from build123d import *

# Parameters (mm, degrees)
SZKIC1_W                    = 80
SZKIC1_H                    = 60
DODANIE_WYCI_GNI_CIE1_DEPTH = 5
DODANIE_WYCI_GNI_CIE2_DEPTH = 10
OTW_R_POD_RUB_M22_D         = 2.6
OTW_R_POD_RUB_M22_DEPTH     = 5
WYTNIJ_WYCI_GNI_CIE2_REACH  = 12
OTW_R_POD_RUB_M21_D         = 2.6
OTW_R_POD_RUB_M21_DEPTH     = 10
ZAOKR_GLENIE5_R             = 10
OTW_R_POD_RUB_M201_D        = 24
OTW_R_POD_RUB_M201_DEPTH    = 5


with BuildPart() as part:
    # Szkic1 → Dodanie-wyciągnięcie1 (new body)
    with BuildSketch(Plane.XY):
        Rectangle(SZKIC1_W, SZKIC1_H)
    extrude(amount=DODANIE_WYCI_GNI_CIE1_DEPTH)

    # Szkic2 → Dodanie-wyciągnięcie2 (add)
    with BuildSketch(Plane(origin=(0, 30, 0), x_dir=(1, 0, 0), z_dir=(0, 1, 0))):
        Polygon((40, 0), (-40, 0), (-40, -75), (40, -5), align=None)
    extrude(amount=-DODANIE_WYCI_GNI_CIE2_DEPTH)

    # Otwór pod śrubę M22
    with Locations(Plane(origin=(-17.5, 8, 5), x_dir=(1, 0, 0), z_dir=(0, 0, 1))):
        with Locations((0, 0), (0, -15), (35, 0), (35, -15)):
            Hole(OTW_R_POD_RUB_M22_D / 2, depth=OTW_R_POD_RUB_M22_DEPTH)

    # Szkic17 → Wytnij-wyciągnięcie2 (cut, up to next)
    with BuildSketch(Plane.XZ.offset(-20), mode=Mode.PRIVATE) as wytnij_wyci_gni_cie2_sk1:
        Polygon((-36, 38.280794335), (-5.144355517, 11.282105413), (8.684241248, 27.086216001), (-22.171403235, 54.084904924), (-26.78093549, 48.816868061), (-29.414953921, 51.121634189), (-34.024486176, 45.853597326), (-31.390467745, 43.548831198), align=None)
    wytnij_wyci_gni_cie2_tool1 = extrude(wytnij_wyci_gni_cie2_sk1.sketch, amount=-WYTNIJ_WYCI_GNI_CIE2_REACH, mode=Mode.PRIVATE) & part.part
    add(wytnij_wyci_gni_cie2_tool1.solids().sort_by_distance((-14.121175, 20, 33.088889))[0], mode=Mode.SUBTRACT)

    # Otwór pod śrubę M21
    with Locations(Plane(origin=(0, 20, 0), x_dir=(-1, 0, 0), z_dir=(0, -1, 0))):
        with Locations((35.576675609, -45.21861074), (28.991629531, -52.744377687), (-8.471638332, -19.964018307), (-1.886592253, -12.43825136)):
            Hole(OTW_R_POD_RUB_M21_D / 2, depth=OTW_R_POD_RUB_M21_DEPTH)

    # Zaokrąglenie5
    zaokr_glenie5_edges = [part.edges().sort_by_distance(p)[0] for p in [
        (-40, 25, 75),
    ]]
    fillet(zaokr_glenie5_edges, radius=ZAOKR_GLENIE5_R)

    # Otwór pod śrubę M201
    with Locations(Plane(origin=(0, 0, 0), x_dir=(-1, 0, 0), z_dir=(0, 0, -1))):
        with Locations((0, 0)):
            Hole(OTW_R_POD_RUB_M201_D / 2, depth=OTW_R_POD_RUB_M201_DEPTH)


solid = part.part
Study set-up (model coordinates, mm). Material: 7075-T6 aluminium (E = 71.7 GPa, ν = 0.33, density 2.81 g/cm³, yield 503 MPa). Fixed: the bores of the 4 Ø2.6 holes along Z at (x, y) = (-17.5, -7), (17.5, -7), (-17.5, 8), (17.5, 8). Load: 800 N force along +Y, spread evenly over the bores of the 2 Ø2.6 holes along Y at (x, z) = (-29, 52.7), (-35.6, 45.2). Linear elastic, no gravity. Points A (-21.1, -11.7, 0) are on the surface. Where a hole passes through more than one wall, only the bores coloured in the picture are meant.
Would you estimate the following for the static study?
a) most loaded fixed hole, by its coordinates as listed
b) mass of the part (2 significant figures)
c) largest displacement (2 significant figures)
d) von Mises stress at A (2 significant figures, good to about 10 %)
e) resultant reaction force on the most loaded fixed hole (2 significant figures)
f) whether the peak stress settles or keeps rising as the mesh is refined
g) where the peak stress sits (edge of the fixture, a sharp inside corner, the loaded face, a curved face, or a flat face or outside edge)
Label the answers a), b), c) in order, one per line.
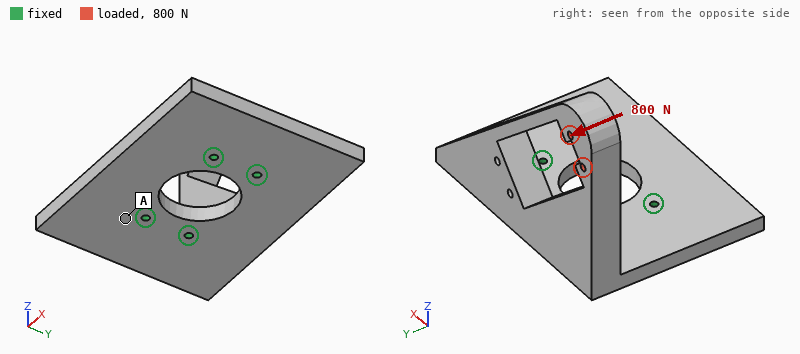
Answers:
a) (-17.5, 8)
b) 110 g
c) 1.1 mm
d) 23 MPa
e) 950 N
f) keeps rising
g) edge of the fixture
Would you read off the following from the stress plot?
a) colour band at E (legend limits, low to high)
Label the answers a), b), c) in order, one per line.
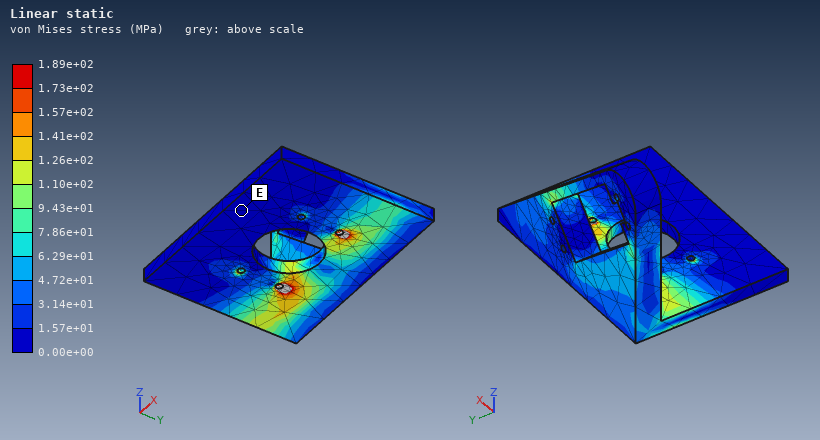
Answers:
a) 0.00e+00 to 1.57e+01 MPa
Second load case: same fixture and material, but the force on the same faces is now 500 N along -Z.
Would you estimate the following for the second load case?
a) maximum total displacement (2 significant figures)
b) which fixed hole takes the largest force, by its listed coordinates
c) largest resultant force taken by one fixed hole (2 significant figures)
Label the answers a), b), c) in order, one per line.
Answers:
a) 0.16 mm
b) (-17.5, 8)
c) 800 N
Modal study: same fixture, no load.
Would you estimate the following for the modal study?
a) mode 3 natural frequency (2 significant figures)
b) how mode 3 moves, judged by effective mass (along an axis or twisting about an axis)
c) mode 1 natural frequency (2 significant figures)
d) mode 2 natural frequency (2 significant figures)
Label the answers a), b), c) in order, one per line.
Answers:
a) 4100 Hz
b) along Z
c) 1200 Hz
d) 2600 Hz
